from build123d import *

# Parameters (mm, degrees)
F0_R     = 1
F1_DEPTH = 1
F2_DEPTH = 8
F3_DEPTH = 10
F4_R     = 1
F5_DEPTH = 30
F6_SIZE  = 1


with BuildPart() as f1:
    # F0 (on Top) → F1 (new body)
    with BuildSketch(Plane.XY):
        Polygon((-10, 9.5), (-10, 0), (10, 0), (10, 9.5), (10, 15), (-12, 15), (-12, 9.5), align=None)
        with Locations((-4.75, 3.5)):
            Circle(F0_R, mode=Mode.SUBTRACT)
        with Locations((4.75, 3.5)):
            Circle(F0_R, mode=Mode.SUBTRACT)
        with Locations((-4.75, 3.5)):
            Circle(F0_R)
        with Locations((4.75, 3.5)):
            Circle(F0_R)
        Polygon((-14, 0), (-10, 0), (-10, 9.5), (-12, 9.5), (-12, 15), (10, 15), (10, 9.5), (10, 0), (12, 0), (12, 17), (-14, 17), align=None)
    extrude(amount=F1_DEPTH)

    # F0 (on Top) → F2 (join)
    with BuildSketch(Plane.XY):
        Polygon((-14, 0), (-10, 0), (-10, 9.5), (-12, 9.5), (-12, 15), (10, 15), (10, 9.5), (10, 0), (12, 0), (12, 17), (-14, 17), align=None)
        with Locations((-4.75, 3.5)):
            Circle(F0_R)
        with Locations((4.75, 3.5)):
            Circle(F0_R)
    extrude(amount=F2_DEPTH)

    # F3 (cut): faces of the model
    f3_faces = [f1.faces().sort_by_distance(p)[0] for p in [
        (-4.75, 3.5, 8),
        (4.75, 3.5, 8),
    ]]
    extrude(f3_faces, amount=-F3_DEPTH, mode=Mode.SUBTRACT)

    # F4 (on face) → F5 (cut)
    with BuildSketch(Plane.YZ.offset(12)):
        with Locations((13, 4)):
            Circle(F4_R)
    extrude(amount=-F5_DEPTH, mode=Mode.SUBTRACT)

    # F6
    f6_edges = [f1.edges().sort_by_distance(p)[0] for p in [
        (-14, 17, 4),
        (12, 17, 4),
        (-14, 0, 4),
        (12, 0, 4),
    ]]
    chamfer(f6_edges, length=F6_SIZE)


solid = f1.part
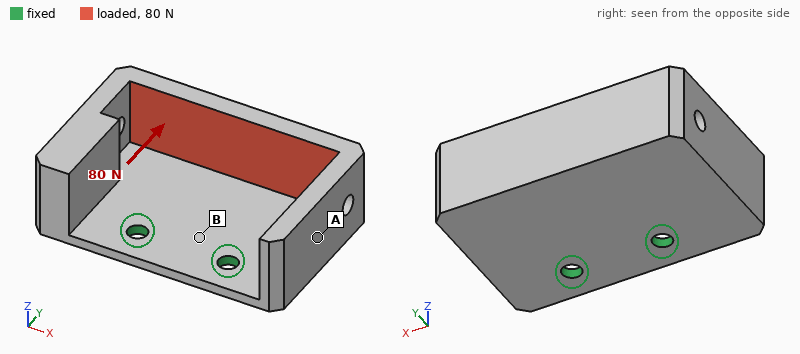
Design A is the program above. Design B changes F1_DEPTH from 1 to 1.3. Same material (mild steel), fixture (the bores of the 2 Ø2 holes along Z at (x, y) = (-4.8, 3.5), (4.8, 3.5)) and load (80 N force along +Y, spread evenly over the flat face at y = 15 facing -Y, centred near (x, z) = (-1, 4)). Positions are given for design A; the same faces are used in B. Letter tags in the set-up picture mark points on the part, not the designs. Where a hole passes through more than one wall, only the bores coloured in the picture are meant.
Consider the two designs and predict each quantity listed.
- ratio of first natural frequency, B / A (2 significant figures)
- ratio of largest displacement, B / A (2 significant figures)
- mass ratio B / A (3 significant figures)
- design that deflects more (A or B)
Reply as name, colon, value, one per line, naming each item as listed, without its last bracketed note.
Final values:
ratio of first natural frequency, B / A: 1.4
ratio of largest displacement, B / A: 0.54
mass ratio B / A: 1.07
design that deflects more: A
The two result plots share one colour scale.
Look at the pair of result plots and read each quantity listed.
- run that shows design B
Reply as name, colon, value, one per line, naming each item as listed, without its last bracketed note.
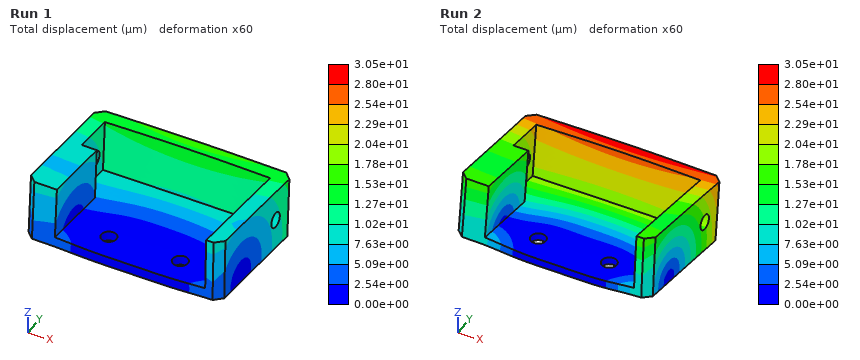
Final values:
run that shows design B: Run 1
